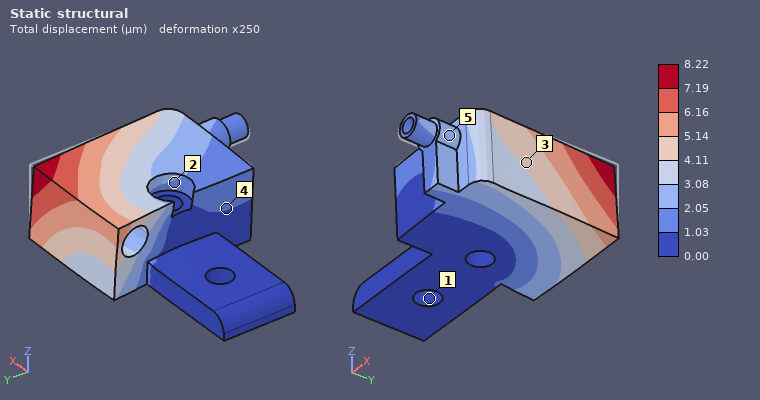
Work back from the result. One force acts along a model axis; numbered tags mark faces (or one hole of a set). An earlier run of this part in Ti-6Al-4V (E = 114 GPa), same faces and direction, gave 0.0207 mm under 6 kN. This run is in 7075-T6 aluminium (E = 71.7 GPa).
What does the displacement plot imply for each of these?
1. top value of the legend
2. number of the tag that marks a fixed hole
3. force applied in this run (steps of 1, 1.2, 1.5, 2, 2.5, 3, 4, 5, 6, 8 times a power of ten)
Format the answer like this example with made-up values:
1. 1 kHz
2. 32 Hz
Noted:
1. 8.22 µm
2. 1
3. 1.5 kN
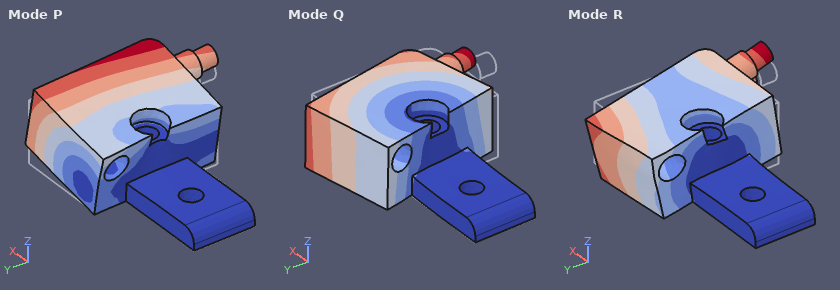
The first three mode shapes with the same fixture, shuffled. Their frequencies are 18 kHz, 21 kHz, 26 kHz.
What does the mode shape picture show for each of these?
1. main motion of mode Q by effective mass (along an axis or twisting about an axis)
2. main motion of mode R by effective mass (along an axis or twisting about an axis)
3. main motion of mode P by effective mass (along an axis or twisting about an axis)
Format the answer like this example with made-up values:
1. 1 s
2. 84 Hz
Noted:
1. along Y
2. twisting about X
3. along Z
